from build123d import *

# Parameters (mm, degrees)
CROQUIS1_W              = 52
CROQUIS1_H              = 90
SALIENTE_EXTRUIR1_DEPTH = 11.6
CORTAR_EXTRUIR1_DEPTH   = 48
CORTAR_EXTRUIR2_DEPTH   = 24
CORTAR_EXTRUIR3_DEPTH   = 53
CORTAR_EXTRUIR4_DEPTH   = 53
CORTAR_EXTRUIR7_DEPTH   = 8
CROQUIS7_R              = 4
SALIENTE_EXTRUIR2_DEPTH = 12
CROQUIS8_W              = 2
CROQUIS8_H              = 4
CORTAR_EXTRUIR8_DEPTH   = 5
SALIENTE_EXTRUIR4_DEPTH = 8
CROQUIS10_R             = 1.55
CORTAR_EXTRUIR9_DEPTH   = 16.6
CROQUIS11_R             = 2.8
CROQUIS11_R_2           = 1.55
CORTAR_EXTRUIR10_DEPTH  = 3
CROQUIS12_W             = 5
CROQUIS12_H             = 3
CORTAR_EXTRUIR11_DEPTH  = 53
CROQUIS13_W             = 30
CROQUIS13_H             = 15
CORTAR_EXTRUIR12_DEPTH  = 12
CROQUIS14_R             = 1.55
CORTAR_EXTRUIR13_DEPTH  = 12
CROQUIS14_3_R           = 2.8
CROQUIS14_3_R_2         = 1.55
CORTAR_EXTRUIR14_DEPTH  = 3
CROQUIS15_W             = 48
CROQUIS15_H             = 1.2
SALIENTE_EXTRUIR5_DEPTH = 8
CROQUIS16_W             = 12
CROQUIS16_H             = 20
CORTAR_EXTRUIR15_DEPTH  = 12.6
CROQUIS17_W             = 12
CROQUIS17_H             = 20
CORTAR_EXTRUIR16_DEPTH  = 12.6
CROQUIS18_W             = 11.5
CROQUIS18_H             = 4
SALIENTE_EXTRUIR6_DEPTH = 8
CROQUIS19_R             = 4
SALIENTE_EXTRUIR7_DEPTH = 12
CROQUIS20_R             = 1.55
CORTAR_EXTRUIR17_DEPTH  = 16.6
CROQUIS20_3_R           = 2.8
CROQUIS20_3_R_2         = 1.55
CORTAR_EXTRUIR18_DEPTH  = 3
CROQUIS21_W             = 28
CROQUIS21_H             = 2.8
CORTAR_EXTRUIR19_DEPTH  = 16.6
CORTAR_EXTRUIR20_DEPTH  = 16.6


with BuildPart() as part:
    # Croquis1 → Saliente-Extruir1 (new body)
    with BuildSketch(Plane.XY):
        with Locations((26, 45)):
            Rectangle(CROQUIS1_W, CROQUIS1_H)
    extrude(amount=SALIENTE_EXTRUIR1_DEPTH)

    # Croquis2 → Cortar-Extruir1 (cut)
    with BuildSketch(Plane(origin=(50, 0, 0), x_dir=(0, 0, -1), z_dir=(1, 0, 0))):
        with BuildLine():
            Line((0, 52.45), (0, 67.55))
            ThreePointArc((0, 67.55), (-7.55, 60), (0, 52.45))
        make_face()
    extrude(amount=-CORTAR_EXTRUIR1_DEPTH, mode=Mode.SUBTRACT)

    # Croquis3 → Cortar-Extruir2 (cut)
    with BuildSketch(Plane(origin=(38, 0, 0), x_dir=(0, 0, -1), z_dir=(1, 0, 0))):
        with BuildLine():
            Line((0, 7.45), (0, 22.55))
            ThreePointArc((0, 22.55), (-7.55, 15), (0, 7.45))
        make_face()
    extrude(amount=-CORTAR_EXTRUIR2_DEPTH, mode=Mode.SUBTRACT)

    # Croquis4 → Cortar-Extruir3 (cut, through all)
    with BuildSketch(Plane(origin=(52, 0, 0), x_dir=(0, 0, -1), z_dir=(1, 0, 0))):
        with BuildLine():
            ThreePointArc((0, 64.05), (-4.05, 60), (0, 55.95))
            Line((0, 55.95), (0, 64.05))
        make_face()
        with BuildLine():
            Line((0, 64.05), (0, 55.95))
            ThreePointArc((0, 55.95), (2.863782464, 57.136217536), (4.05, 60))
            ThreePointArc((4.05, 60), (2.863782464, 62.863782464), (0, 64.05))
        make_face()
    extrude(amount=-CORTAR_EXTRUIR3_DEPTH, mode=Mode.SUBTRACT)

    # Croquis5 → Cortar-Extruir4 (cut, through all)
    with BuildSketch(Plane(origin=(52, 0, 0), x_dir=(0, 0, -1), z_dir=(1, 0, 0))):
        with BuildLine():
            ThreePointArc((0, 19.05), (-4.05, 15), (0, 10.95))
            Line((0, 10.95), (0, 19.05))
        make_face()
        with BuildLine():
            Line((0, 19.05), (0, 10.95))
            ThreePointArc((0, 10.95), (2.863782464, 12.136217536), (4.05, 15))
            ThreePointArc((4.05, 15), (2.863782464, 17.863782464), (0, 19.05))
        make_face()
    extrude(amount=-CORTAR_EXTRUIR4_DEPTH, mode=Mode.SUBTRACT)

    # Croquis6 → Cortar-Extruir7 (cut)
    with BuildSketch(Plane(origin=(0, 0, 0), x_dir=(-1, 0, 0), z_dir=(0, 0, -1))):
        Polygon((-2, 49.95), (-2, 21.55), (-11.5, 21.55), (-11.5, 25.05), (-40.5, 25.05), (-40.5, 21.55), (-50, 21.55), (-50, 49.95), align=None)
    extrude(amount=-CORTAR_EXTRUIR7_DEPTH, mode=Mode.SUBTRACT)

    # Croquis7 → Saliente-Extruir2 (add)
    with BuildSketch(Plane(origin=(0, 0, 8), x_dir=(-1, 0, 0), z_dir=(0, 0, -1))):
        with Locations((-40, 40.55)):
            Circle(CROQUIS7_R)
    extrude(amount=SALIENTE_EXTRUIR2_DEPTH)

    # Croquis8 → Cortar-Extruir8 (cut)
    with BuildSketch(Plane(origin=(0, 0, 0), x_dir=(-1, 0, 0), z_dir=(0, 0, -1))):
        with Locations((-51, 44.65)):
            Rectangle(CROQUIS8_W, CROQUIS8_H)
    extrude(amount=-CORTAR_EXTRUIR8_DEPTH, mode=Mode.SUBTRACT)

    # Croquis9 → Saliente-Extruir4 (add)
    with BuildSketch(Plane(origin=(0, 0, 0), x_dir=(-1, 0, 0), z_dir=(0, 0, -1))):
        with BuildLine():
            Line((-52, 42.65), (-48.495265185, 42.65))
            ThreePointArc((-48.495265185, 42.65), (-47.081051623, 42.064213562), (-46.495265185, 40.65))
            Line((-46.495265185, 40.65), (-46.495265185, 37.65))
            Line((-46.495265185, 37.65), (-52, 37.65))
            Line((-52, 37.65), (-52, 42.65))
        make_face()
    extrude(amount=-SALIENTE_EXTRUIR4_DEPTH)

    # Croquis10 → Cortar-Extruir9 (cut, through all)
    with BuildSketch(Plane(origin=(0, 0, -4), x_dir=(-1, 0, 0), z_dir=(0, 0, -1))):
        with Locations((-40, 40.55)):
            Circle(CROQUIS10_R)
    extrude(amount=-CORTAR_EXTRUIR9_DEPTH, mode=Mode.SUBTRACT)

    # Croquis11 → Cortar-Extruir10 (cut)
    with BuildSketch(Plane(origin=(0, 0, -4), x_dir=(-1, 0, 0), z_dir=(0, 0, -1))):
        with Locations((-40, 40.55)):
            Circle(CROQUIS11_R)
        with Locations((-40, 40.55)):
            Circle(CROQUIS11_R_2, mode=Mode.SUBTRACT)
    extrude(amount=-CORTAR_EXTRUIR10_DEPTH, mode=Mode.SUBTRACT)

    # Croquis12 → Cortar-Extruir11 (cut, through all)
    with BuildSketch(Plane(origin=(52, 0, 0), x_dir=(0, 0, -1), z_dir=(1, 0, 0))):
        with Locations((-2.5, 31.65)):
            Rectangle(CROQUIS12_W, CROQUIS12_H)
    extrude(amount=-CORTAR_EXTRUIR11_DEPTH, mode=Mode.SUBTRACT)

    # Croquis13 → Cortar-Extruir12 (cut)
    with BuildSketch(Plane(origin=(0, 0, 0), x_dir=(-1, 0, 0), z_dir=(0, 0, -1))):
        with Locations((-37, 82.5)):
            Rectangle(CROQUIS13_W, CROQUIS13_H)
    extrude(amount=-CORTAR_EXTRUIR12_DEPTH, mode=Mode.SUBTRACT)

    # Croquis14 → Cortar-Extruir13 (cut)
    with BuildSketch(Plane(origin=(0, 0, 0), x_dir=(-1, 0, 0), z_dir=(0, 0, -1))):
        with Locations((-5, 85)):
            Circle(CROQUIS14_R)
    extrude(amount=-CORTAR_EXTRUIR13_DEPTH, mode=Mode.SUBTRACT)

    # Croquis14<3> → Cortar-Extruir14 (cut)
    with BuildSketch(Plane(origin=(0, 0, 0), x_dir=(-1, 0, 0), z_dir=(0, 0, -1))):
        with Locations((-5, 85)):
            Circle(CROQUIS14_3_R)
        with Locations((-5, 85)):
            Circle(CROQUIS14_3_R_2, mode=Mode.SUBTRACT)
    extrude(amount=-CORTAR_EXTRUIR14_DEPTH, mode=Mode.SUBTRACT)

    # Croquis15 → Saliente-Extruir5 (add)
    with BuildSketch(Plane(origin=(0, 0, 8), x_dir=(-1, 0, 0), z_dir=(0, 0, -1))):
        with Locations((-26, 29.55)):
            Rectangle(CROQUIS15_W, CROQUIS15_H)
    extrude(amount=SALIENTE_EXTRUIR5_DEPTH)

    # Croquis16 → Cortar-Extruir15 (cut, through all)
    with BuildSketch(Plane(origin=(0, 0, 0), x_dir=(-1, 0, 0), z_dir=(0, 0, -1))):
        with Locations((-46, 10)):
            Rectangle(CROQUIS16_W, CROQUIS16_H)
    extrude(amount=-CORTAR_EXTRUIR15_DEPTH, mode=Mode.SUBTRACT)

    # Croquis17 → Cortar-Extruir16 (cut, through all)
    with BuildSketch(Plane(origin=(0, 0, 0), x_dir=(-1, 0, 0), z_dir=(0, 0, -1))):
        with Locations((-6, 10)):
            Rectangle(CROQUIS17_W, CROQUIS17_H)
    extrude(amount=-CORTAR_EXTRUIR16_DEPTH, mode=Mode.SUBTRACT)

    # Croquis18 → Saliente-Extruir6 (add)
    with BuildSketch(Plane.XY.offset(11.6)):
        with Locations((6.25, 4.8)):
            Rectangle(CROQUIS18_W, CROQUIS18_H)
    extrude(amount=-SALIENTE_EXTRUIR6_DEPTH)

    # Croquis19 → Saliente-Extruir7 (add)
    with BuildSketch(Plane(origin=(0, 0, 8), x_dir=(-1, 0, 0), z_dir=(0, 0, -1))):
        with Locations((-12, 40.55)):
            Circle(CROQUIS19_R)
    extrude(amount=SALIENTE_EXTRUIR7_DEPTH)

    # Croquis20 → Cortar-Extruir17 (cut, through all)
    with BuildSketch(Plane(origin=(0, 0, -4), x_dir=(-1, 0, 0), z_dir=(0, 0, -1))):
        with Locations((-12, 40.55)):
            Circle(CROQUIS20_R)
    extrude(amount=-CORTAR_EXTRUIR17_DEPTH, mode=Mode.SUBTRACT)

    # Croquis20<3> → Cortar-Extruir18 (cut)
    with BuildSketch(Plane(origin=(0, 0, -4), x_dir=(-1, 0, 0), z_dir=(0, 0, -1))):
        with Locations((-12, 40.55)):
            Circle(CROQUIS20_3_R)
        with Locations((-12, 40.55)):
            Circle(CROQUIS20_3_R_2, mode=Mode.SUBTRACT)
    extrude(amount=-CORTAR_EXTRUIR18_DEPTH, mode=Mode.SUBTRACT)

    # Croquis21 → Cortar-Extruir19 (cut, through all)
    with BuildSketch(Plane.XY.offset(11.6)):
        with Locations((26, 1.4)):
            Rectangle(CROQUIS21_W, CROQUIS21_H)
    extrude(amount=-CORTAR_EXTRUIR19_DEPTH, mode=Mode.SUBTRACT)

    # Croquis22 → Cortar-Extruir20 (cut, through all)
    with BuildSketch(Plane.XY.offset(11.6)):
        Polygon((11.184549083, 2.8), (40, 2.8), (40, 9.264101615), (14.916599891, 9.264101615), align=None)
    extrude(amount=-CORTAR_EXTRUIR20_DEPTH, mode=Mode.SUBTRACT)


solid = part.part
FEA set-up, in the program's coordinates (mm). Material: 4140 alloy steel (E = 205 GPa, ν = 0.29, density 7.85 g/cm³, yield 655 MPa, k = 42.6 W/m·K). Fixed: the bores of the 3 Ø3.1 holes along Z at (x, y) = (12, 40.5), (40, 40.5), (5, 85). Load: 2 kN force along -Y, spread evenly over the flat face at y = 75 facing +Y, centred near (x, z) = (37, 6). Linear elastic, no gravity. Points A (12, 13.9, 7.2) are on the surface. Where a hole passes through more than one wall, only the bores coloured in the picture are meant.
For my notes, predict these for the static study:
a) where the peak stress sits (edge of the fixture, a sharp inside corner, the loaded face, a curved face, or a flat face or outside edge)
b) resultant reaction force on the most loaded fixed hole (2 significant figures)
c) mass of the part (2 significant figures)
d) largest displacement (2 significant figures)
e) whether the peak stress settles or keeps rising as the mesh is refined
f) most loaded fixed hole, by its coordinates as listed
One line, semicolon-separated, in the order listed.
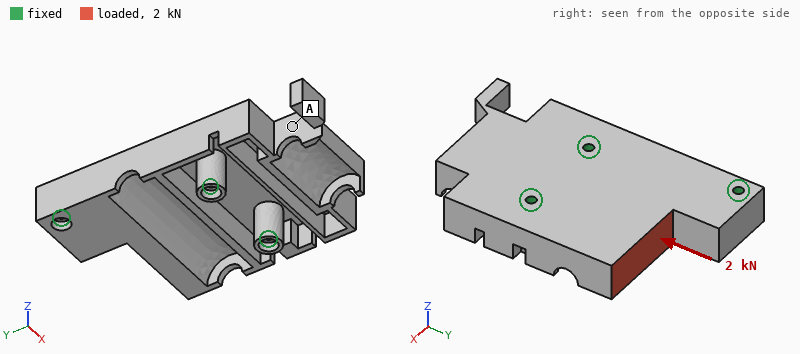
edge of the fixture; 1.1 kN; 200 g; 14 µm; keeps rising; (40, 40.5)
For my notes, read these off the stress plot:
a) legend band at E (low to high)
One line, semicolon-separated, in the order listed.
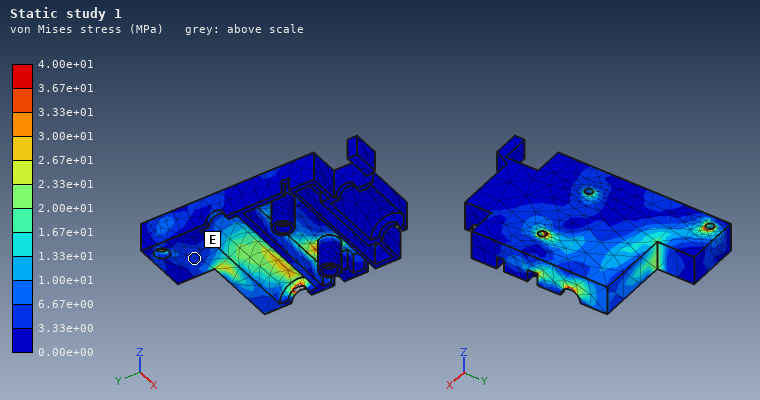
3.33e+00 to 6.67e+00 MPa
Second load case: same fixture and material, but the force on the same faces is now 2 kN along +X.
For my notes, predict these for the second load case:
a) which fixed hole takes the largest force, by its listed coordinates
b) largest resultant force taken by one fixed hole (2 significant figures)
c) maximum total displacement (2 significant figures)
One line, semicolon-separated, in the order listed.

(5, 85); 1.2 kN; 7.1 µm
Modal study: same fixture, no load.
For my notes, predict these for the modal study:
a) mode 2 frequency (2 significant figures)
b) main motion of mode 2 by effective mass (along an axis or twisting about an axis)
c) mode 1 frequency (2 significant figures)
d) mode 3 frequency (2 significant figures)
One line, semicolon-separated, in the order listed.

5000 Hz; along Z; 2900 Hz; 5200 Hz
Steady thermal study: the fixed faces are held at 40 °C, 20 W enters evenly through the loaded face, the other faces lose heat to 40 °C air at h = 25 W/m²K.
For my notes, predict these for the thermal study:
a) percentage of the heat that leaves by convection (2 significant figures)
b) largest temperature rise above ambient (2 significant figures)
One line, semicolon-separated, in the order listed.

17 %; 56 K
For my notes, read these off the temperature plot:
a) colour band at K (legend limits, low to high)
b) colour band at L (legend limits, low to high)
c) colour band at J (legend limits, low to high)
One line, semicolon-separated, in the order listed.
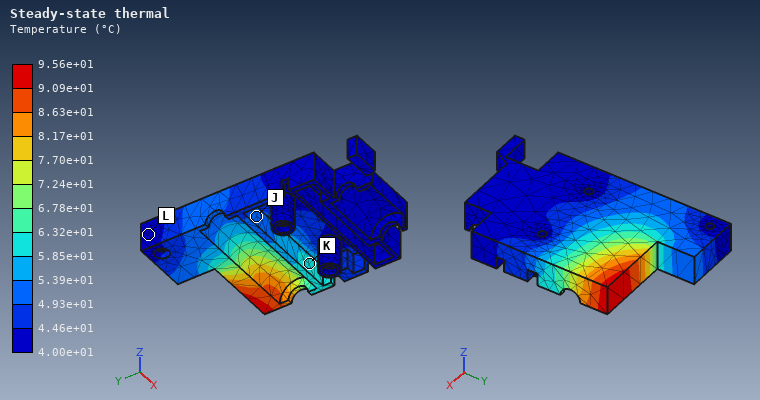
5.85e+01 to 6.32e+01 °C; 4.00e+01 to 4.46e+01 °C; 4.93e+01 to 5.39e+01 °C
